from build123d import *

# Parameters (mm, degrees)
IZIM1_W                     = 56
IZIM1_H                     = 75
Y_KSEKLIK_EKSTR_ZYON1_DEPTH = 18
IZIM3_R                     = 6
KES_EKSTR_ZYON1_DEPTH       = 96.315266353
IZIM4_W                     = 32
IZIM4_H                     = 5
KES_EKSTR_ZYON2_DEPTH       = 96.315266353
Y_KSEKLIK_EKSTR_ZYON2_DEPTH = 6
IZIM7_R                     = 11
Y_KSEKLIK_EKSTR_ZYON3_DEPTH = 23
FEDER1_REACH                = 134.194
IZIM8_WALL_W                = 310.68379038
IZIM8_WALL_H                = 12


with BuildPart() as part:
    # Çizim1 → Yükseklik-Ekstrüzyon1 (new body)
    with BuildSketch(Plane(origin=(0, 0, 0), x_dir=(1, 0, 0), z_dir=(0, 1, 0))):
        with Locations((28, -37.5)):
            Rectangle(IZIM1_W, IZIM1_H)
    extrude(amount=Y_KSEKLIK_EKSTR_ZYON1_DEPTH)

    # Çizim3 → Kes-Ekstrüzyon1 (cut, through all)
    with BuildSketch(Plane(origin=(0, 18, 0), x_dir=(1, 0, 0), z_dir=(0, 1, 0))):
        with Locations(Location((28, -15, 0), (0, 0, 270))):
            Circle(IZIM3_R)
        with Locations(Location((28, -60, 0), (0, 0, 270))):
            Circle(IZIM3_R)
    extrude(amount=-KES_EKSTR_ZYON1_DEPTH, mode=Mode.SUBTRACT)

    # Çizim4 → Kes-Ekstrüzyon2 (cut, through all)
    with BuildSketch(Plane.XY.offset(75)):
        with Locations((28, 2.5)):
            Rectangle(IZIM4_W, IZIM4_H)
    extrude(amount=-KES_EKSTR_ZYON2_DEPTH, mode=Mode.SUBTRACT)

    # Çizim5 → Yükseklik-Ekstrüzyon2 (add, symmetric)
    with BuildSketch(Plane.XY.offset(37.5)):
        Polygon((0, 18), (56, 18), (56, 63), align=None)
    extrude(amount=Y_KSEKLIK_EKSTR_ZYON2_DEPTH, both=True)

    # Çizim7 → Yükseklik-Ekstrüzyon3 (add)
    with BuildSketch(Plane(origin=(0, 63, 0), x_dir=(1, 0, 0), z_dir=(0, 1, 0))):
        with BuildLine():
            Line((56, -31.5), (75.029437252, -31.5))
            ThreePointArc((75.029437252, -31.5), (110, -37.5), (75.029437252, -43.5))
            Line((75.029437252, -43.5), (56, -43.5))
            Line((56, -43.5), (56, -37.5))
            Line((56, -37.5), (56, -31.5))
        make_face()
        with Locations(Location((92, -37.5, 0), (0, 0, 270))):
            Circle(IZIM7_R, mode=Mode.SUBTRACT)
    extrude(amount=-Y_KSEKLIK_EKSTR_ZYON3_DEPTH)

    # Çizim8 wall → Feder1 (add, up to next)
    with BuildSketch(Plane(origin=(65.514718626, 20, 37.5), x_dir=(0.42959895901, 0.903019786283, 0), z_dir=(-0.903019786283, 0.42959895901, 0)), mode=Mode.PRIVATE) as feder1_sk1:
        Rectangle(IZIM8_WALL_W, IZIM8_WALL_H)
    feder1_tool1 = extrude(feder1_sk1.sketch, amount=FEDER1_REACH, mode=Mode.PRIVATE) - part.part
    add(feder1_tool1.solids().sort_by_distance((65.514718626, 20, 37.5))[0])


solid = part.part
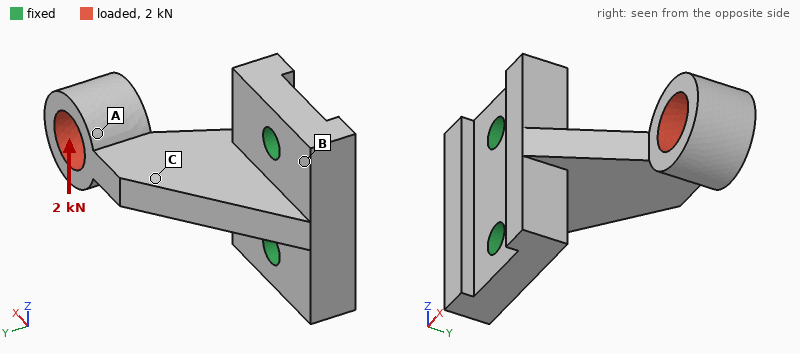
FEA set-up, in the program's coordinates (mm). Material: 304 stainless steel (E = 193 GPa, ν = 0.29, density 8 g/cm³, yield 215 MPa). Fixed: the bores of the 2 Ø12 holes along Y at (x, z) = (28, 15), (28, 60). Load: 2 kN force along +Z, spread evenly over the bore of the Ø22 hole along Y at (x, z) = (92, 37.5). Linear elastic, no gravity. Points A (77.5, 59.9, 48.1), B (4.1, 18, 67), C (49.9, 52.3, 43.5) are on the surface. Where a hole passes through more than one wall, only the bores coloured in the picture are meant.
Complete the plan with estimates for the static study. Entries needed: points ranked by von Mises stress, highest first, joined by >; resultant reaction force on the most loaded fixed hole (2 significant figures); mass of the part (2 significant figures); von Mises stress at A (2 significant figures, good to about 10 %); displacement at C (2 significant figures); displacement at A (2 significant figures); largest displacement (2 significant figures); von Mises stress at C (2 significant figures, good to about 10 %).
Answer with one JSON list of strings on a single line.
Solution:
["C > A > B", "3.4 kN", "800 g", "30 MPa", "0.044 mm", "0.13 mm", "0.25 mm", "67 MPa"]
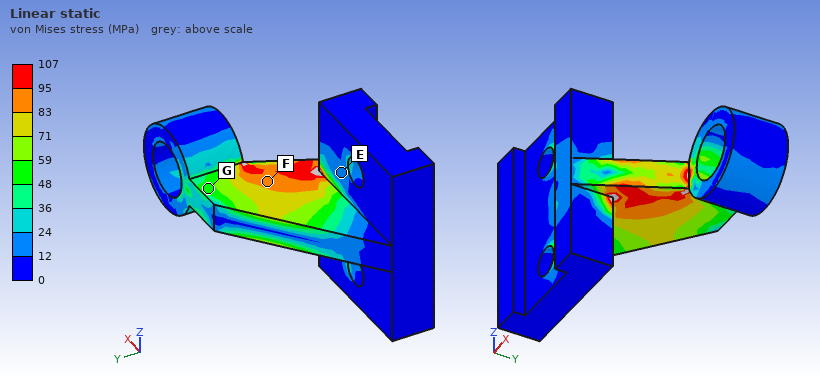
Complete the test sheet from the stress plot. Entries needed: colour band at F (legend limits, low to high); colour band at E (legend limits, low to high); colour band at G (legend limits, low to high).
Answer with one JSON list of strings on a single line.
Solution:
["83 to 95 MPa", "12 to 24 MPa", "48 to 59 MPa"]
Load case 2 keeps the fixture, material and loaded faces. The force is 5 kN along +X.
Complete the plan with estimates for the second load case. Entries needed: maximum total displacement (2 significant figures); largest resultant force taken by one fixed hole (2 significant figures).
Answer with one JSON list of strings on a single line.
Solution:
["84 µm", "2.5 kN"]
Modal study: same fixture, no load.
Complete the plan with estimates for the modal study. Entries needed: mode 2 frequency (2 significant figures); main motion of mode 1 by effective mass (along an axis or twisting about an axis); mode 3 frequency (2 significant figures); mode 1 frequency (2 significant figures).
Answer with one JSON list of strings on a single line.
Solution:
["2400 Hz", "along Z", "3900 Hz", "1500 Hz"]
